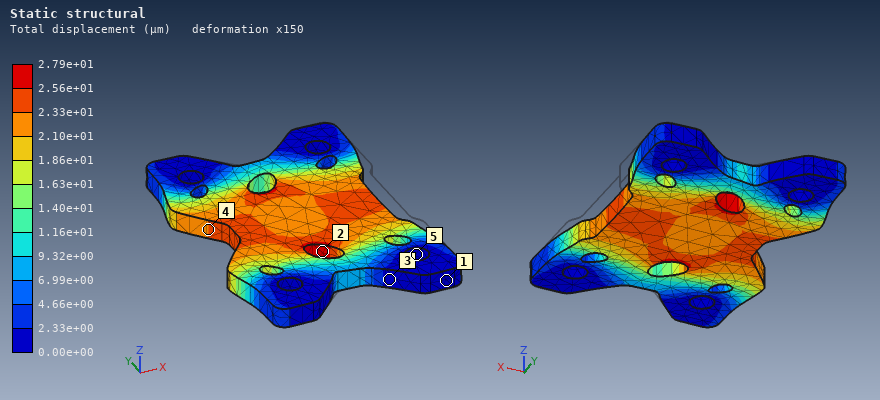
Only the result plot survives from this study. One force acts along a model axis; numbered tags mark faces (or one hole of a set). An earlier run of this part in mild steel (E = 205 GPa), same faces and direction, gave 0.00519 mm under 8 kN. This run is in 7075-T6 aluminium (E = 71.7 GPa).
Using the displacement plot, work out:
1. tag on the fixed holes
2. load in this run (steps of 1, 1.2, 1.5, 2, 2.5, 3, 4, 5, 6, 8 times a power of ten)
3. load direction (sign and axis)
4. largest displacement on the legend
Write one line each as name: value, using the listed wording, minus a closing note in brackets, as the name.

tag on the fixed holes: 5
load in this run: 15 kN
load direction: -X
largest displacement on the legend: 2.79e+01 µm
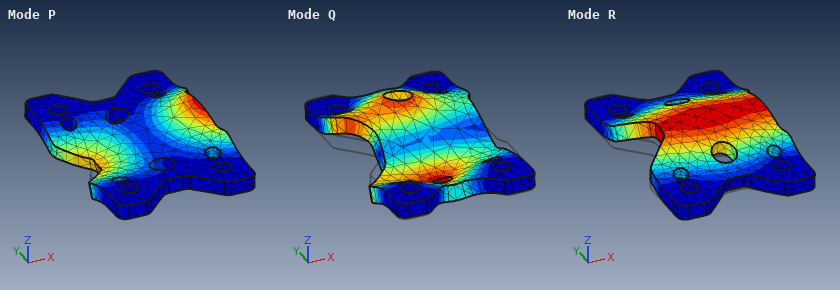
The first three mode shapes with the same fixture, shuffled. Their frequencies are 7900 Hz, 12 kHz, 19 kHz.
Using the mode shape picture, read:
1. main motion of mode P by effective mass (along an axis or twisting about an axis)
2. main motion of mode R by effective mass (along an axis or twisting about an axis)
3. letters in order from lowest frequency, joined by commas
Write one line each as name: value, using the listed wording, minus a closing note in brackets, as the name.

main motion of mode P by effective mass: twisting about Y
main motion of mode R by effective mass: along Z
letters in order from lowest frequency, joined by commas: R, P, Q
